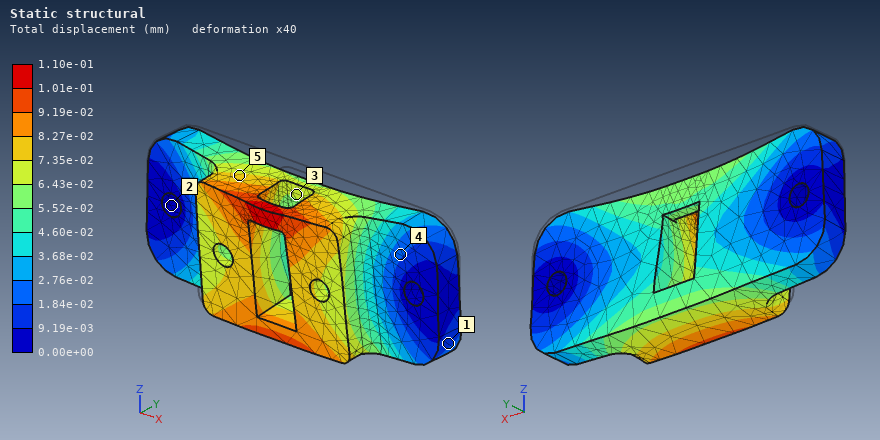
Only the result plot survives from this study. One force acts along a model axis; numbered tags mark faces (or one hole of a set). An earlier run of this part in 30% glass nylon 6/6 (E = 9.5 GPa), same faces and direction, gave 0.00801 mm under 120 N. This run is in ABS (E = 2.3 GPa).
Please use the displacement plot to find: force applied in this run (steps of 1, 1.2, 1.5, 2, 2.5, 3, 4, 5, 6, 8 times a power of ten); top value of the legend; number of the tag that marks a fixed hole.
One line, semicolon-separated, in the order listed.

400 N; 1.10e-01 mm; 2
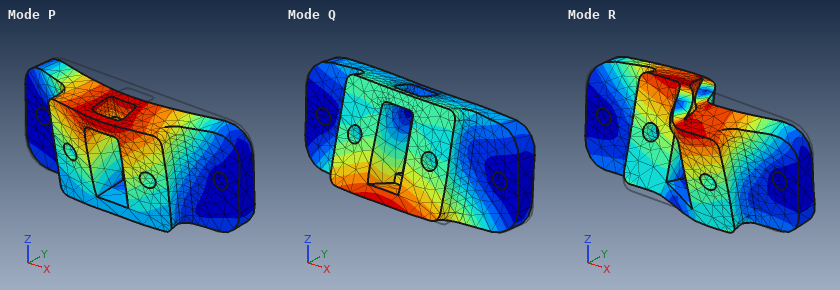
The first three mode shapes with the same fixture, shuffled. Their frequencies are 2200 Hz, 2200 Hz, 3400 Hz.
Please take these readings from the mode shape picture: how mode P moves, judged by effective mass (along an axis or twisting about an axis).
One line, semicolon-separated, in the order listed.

along Y
